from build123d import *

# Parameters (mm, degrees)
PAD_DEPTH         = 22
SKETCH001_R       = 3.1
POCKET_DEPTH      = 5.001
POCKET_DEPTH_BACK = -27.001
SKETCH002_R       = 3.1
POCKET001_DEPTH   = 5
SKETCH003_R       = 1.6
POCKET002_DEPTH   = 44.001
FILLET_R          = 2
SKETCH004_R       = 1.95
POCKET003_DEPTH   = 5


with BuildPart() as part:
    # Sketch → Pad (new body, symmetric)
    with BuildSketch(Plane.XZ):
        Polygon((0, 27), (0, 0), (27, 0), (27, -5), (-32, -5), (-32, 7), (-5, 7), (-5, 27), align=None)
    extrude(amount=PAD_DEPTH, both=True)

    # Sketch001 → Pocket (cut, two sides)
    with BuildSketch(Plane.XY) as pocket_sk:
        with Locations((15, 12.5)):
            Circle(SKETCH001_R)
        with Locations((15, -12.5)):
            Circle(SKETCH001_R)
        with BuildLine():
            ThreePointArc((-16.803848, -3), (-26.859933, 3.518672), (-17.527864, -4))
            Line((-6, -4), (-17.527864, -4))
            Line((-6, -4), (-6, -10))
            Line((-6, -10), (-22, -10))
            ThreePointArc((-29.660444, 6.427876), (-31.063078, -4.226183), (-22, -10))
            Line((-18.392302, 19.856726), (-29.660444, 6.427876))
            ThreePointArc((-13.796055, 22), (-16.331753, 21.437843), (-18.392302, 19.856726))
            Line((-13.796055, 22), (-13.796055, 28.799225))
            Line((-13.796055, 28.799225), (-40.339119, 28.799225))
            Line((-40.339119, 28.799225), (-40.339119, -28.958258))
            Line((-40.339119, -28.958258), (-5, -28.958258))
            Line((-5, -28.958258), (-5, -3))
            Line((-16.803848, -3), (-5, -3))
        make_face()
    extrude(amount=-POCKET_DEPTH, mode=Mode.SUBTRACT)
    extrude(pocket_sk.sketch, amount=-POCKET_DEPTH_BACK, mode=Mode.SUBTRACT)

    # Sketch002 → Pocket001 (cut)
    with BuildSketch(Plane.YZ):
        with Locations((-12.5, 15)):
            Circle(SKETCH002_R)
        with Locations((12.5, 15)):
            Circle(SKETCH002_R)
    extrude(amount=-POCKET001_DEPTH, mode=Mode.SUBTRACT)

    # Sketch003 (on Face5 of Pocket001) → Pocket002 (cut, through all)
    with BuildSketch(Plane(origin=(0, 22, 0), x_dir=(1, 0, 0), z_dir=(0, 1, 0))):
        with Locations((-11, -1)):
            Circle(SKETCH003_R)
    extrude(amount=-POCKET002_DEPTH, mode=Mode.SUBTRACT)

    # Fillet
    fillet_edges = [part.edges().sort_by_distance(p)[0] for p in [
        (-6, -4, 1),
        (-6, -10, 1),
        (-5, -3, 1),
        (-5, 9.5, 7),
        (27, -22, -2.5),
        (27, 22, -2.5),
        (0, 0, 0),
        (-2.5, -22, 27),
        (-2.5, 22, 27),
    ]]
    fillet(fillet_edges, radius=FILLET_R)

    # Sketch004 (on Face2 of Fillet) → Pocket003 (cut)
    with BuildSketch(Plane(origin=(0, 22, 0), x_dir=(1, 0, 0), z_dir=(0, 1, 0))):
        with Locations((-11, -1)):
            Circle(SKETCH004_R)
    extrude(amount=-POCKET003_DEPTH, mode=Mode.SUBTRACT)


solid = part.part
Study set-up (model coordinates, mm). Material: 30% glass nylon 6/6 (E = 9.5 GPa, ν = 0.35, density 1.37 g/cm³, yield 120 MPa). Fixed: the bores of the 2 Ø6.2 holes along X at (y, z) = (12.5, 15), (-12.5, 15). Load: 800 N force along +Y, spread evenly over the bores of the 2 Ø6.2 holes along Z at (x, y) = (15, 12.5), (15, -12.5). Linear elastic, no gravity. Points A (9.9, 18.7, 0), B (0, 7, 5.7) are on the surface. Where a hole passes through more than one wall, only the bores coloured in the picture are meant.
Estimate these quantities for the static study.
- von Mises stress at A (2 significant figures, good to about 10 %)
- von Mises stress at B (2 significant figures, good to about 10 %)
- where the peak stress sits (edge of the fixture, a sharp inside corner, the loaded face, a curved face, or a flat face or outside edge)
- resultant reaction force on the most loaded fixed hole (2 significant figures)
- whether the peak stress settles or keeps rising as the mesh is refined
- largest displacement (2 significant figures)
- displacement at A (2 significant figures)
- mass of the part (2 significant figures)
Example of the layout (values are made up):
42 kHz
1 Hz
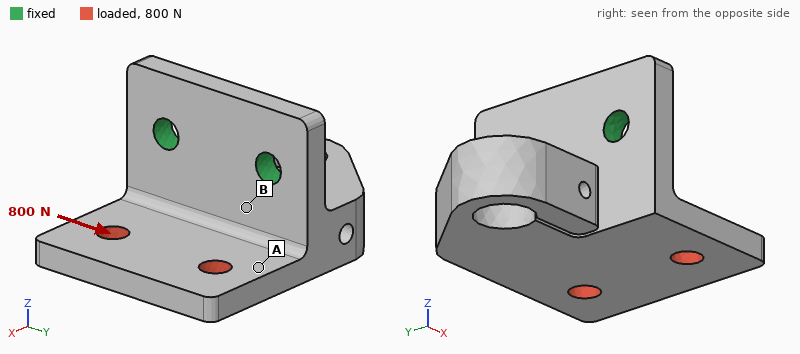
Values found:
11 MPa
24 MPa
edge of the fixture
770 N
keeps rising
0.33 mm
0.19 mm
26 g
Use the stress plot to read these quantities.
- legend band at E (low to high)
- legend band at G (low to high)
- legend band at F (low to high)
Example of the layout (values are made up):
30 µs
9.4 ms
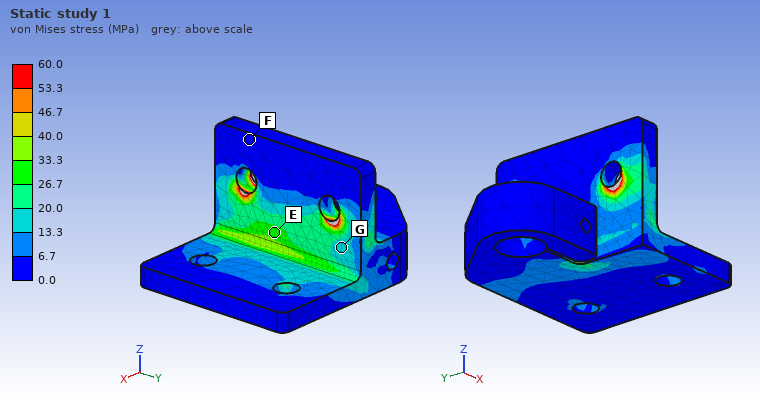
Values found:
26.7 to 33.3 MPa
13.3 to 20.0 MPa
0.0 to 6.7 MPa
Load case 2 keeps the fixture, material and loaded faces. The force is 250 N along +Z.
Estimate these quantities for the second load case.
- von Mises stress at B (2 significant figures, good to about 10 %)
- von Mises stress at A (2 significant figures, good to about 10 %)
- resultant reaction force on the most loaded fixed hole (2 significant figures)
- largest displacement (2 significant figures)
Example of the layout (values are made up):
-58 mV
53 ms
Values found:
16 MPa
7.7 MPa
130 N
0.51 mm
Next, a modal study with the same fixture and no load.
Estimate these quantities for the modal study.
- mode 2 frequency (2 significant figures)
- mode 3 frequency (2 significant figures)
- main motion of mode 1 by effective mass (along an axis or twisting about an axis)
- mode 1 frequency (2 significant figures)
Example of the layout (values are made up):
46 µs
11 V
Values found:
1300 Hz
1600 Hz
along X
1200 Hz
